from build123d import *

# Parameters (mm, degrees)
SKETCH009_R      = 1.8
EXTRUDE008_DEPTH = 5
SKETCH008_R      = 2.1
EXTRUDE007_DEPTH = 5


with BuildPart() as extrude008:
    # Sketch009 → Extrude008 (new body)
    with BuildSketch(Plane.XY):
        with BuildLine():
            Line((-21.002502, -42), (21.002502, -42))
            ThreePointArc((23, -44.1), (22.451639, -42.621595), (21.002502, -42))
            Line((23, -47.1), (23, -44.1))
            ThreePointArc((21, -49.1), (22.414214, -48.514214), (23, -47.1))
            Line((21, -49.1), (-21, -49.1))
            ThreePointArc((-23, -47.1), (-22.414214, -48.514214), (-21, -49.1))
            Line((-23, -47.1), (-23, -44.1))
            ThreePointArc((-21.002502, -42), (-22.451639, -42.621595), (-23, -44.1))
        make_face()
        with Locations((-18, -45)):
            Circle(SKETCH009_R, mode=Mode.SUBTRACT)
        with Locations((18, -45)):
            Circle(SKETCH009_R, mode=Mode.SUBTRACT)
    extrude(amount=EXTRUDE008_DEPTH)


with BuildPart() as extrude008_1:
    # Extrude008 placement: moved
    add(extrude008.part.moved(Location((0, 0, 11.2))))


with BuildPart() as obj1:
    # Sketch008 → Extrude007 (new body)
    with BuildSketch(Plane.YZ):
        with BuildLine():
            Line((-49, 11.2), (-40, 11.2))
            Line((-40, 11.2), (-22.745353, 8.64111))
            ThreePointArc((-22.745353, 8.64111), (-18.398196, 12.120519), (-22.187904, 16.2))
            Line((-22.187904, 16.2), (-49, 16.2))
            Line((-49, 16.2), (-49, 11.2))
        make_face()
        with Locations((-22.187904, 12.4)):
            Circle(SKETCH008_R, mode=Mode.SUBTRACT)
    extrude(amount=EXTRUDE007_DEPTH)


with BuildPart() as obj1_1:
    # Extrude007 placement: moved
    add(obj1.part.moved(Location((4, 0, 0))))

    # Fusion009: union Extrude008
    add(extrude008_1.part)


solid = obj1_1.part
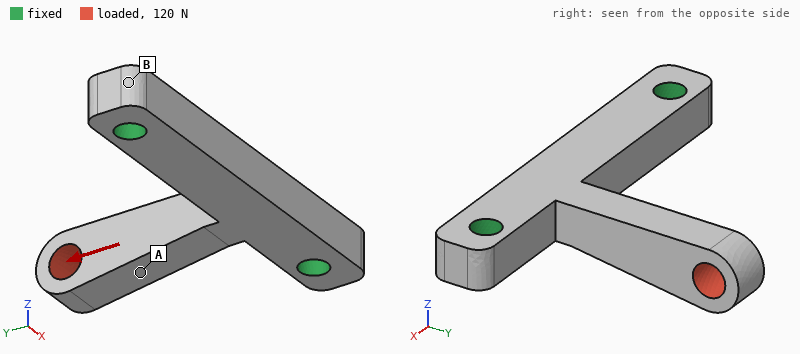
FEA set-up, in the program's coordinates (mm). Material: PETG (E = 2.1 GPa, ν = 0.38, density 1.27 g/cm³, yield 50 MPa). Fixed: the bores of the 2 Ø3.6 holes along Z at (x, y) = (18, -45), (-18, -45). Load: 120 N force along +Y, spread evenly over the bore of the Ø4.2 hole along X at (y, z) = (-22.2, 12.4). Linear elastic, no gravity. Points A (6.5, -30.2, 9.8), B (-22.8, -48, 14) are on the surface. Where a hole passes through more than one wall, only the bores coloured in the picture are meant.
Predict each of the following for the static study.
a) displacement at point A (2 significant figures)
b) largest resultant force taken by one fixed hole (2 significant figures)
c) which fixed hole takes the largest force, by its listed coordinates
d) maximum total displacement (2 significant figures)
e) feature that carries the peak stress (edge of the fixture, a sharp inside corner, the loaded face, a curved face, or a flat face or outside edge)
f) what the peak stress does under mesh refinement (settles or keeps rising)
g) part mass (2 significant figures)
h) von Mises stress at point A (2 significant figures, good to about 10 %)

0.31 mm
89 N
(18, -45)
0.54 mm
edge of the fixture
keeps rising
2.8 g
5.8 MPa
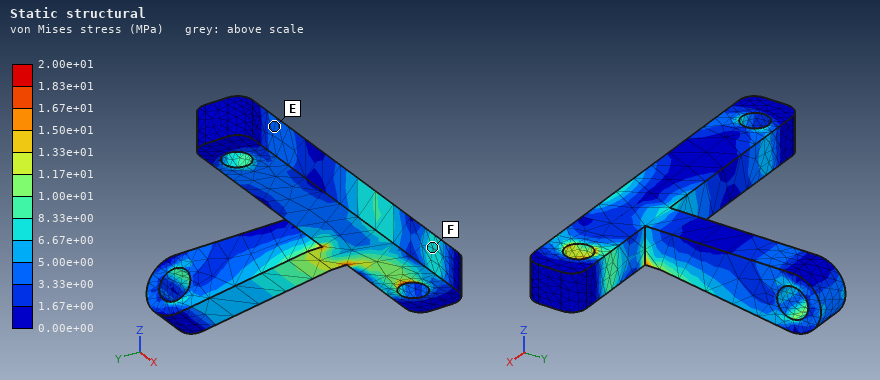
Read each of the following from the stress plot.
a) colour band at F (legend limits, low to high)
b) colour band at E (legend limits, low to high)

6.67e+00 to 8.33e+00 MPa
3.33e+00 to 5.00e+00 MPa
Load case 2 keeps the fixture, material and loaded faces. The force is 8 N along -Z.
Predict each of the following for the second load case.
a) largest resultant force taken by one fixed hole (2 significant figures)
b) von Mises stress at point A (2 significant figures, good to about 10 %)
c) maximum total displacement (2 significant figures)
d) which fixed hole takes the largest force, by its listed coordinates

6.7 N
1.7 MPa
0.54 mm
(18, -45)
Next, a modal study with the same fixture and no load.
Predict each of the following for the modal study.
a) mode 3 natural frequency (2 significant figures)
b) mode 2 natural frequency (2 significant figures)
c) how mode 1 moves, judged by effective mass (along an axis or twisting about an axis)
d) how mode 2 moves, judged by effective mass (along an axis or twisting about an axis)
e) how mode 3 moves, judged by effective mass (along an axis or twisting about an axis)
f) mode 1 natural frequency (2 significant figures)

4400 Hz
1500 Hz
along Z
along X
along Y
1100 Hz
